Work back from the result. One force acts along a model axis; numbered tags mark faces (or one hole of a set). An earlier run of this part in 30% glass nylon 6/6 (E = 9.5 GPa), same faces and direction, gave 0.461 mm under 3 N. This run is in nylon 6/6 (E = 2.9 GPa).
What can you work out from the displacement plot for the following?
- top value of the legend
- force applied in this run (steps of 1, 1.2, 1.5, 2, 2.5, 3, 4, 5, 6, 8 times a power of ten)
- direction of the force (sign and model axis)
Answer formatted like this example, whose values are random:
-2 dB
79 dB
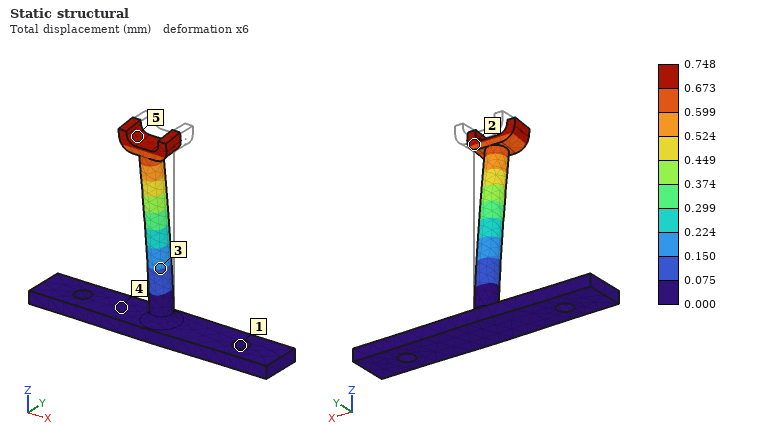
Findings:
0.748 mm
1.5 N
-Y
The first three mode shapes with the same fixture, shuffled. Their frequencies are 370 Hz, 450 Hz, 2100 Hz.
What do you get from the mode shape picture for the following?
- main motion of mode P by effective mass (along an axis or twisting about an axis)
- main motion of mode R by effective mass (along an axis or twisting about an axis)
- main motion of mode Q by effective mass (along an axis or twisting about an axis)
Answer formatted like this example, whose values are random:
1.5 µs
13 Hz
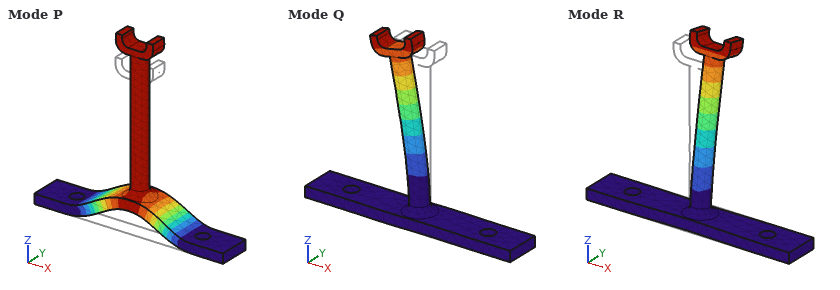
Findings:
along Z
along Y
along X
